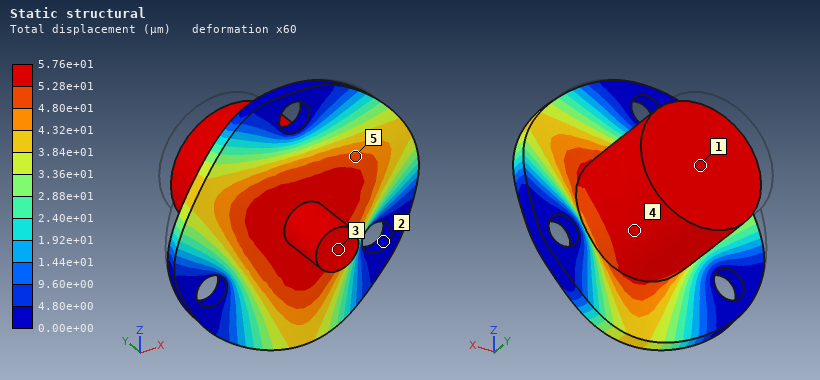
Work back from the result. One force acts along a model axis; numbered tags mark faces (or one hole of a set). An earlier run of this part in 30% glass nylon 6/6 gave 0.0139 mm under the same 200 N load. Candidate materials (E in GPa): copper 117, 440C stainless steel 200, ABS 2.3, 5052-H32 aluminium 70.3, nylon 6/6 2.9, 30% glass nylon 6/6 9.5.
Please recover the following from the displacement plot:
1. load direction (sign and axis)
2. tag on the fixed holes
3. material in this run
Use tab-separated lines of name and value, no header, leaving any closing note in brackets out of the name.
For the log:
load direction	-Y
tag on the fixed holes	2
material in this run	ABS
